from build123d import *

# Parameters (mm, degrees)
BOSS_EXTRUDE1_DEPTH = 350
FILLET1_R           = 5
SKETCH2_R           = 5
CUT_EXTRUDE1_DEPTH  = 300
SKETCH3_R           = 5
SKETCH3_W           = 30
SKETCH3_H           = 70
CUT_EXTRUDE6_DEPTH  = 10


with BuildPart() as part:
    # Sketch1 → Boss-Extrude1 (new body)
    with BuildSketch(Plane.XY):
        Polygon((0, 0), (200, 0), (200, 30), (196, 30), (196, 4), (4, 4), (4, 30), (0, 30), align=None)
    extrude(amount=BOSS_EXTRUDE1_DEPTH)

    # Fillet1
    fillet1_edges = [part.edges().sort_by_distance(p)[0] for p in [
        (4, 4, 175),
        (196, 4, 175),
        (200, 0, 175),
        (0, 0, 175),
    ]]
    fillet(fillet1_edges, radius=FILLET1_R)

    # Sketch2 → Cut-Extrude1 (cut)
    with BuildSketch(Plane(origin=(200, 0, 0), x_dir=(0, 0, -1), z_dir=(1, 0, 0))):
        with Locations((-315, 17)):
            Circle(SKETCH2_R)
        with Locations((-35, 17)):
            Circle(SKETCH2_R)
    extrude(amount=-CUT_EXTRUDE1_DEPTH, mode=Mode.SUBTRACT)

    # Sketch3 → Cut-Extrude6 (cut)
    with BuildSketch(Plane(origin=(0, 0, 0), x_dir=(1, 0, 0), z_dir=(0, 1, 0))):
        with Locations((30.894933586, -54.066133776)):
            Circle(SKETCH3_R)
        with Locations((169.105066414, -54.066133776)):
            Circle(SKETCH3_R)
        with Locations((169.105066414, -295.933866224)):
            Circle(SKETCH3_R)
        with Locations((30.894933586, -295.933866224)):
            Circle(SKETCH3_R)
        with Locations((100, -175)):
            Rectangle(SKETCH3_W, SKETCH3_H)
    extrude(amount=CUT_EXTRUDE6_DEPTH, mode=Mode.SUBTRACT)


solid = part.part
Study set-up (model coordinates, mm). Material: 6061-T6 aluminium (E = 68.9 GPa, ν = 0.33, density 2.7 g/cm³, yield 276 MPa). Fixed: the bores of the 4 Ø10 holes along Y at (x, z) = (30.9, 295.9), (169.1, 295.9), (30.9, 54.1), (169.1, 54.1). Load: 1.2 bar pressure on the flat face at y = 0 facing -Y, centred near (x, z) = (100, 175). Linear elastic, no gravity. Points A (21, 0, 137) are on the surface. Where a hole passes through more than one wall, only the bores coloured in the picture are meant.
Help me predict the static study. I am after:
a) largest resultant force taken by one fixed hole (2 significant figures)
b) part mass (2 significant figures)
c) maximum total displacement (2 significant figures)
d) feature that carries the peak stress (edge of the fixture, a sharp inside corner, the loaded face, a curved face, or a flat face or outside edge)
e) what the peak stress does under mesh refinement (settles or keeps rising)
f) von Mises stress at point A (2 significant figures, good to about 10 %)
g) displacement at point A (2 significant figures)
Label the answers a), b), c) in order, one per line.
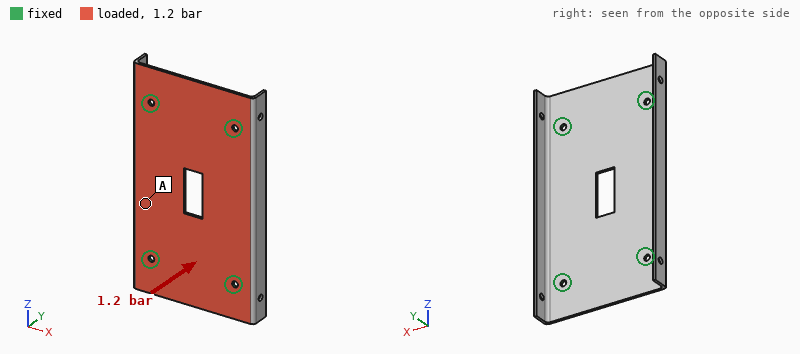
a) 2.1 kN
b) 920 g
c) 2.1 mm
d) edge of the fixture
e) keeps rising
f) 34 MPa
g) 0.51 mm
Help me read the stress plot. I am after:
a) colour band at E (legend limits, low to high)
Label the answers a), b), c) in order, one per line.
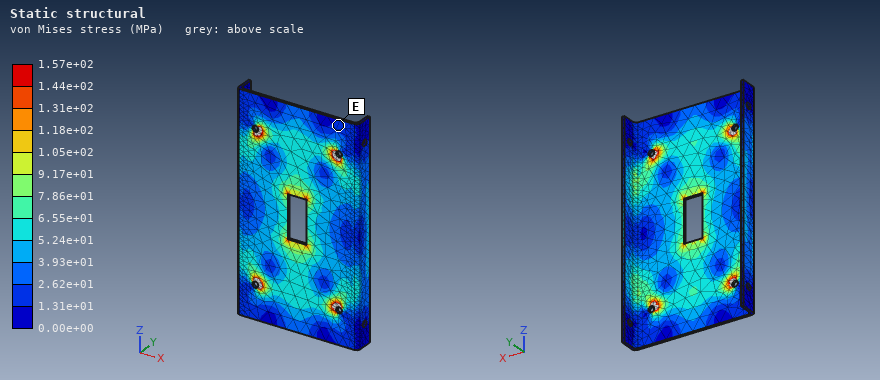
a) 1.31e+01 to 2.62e+01 MPa
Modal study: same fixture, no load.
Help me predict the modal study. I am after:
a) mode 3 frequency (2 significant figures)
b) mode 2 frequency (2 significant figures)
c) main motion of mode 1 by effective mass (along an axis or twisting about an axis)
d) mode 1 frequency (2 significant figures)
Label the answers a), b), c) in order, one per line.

a) 850 Hz
b) 800 Hz
c) along Y
d) 480 Hz
